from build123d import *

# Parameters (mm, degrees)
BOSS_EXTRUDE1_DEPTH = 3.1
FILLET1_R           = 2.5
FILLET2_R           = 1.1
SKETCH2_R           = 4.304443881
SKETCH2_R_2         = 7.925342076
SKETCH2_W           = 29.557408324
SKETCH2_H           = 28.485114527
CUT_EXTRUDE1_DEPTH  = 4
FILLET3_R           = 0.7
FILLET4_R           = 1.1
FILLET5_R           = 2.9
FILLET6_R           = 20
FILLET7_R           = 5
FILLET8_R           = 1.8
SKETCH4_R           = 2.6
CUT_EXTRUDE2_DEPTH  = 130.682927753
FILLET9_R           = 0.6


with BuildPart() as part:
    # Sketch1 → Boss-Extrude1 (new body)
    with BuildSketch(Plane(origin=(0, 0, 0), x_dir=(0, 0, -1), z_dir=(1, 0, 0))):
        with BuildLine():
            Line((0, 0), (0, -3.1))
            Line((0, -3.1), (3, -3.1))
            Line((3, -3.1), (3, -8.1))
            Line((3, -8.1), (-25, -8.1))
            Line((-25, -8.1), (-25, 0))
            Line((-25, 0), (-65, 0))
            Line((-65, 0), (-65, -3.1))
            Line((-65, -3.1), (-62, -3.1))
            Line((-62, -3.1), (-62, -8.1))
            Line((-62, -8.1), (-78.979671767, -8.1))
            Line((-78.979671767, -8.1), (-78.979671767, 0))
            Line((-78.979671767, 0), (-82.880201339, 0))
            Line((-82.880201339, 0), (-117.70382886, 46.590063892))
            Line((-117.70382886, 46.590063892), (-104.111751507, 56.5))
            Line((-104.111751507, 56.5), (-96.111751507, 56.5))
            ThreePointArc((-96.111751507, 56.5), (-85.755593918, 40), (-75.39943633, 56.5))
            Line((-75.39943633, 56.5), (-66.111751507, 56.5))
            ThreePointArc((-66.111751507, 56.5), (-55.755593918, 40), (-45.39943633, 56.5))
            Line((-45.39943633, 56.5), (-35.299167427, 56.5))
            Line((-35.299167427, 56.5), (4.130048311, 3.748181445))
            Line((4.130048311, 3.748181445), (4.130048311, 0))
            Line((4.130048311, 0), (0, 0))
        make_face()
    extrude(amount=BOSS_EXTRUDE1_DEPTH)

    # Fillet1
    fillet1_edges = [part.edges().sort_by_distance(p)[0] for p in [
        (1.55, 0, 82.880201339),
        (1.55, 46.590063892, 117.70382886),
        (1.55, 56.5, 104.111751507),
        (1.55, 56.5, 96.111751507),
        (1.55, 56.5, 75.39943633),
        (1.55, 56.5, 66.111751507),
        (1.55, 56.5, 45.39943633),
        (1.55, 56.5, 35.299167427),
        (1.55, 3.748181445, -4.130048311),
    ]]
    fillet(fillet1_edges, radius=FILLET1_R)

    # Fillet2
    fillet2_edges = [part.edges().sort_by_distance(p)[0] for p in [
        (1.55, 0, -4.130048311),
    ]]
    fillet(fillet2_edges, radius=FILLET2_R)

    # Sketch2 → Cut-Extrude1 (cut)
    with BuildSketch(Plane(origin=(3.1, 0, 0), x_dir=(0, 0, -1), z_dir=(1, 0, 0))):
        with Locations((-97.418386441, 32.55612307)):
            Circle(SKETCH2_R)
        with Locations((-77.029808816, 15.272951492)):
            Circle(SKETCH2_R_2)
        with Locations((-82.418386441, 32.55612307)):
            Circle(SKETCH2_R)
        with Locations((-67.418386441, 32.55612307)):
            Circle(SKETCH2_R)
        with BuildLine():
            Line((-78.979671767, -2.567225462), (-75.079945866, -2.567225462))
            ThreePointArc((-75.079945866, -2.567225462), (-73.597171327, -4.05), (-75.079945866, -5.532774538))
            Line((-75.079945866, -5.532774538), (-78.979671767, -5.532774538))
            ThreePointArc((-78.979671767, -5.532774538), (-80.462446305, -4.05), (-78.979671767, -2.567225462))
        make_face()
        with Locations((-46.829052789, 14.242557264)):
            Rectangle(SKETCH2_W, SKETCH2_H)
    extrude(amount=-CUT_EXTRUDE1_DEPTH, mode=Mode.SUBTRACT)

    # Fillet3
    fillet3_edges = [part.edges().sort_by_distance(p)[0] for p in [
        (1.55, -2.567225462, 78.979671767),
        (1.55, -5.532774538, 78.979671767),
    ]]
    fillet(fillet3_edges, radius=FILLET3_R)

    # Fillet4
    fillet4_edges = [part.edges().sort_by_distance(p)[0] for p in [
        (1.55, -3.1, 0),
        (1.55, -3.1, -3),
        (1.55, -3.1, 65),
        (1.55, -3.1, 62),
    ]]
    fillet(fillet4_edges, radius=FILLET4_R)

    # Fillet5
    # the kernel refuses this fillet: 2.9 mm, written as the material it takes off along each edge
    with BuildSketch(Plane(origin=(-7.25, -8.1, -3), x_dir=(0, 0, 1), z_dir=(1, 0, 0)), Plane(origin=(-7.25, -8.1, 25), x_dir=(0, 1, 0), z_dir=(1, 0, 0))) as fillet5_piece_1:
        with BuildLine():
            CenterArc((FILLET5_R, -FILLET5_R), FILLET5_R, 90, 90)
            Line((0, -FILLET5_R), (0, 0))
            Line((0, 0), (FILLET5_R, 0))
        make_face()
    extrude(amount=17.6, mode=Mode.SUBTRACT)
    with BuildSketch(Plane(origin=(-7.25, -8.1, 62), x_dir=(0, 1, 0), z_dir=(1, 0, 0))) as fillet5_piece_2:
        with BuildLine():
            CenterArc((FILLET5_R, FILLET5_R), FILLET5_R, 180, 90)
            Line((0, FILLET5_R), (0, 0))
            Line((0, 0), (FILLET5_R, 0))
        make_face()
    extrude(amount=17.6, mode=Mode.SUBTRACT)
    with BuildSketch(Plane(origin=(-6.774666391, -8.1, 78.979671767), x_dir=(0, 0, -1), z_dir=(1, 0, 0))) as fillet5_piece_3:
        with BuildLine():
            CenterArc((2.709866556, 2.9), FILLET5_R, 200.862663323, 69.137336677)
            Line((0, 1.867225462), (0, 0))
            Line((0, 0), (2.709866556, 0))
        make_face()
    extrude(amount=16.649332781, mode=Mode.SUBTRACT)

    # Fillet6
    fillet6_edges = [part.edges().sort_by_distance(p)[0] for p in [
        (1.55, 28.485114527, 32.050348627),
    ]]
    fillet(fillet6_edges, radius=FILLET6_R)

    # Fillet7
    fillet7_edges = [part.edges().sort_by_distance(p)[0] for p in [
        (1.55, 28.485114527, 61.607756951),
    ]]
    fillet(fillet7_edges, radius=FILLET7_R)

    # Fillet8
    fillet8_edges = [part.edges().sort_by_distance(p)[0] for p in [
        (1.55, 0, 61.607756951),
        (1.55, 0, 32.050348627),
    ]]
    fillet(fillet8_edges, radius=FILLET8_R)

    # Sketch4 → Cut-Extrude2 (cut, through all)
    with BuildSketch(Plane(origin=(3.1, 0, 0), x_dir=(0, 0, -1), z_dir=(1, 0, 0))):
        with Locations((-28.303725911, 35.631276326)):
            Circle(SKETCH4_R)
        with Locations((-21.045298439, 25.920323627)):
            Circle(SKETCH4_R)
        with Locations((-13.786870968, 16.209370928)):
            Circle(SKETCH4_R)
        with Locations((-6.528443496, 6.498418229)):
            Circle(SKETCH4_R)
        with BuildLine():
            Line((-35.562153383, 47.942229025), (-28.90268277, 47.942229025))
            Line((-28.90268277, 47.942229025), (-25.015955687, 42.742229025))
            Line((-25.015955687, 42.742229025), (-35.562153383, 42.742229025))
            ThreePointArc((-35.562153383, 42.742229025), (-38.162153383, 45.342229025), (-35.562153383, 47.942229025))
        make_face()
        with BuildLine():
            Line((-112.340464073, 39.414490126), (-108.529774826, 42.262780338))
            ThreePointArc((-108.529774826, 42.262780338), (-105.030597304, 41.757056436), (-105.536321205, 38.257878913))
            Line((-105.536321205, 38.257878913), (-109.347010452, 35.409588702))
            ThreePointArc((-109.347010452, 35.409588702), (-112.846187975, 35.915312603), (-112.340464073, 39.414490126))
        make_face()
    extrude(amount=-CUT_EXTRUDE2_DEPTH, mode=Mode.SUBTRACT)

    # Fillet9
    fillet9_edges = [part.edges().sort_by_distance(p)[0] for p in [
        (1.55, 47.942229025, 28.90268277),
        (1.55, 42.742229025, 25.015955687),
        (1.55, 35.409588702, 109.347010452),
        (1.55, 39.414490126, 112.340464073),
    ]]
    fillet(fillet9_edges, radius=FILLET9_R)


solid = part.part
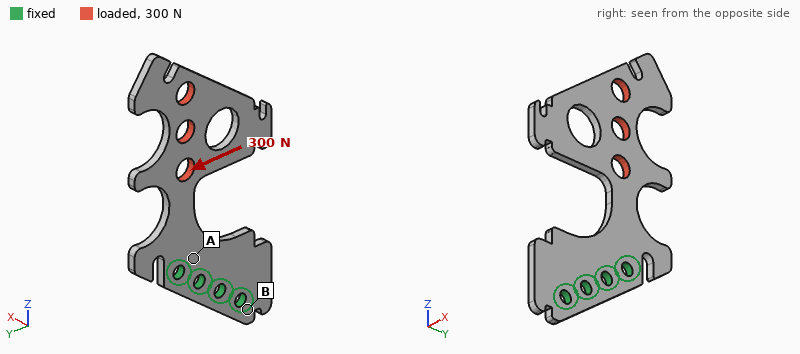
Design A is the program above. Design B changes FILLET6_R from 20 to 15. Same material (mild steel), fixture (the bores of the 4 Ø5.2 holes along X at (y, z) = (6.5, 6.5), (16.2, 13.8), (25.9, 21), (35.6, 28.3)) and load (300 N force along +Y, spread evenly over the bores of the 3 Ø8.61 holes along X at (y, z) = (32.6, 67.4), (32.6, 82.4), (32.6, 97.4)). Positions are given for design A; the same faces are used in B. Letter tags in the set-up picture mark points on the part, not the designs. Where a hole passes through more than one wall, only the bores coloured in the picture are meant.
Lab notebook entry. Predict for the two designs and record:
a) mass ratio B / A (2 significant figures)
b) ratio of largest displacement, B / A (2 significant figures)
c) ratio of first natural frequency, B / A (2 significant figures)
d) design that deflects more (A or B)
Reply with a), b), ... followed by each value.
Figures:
a) 0.99
b) 1.1
c) 0.98
d) B
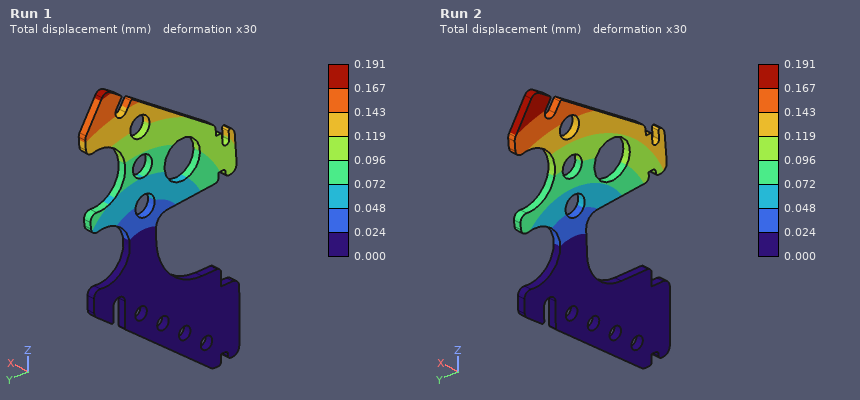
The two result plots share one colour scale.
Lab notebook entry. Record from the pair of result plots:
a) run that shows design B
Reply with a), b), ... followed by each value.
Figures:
a) Run 2
